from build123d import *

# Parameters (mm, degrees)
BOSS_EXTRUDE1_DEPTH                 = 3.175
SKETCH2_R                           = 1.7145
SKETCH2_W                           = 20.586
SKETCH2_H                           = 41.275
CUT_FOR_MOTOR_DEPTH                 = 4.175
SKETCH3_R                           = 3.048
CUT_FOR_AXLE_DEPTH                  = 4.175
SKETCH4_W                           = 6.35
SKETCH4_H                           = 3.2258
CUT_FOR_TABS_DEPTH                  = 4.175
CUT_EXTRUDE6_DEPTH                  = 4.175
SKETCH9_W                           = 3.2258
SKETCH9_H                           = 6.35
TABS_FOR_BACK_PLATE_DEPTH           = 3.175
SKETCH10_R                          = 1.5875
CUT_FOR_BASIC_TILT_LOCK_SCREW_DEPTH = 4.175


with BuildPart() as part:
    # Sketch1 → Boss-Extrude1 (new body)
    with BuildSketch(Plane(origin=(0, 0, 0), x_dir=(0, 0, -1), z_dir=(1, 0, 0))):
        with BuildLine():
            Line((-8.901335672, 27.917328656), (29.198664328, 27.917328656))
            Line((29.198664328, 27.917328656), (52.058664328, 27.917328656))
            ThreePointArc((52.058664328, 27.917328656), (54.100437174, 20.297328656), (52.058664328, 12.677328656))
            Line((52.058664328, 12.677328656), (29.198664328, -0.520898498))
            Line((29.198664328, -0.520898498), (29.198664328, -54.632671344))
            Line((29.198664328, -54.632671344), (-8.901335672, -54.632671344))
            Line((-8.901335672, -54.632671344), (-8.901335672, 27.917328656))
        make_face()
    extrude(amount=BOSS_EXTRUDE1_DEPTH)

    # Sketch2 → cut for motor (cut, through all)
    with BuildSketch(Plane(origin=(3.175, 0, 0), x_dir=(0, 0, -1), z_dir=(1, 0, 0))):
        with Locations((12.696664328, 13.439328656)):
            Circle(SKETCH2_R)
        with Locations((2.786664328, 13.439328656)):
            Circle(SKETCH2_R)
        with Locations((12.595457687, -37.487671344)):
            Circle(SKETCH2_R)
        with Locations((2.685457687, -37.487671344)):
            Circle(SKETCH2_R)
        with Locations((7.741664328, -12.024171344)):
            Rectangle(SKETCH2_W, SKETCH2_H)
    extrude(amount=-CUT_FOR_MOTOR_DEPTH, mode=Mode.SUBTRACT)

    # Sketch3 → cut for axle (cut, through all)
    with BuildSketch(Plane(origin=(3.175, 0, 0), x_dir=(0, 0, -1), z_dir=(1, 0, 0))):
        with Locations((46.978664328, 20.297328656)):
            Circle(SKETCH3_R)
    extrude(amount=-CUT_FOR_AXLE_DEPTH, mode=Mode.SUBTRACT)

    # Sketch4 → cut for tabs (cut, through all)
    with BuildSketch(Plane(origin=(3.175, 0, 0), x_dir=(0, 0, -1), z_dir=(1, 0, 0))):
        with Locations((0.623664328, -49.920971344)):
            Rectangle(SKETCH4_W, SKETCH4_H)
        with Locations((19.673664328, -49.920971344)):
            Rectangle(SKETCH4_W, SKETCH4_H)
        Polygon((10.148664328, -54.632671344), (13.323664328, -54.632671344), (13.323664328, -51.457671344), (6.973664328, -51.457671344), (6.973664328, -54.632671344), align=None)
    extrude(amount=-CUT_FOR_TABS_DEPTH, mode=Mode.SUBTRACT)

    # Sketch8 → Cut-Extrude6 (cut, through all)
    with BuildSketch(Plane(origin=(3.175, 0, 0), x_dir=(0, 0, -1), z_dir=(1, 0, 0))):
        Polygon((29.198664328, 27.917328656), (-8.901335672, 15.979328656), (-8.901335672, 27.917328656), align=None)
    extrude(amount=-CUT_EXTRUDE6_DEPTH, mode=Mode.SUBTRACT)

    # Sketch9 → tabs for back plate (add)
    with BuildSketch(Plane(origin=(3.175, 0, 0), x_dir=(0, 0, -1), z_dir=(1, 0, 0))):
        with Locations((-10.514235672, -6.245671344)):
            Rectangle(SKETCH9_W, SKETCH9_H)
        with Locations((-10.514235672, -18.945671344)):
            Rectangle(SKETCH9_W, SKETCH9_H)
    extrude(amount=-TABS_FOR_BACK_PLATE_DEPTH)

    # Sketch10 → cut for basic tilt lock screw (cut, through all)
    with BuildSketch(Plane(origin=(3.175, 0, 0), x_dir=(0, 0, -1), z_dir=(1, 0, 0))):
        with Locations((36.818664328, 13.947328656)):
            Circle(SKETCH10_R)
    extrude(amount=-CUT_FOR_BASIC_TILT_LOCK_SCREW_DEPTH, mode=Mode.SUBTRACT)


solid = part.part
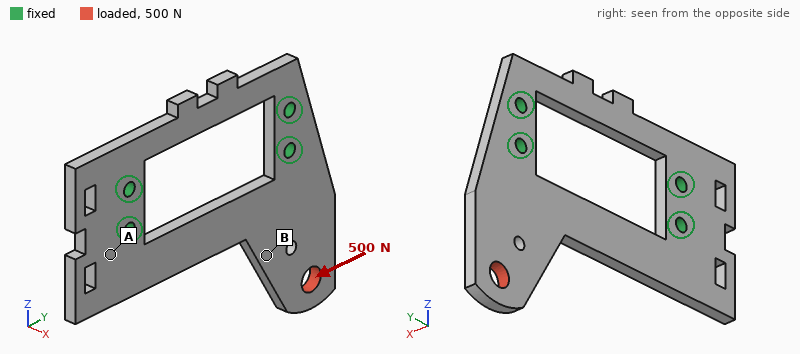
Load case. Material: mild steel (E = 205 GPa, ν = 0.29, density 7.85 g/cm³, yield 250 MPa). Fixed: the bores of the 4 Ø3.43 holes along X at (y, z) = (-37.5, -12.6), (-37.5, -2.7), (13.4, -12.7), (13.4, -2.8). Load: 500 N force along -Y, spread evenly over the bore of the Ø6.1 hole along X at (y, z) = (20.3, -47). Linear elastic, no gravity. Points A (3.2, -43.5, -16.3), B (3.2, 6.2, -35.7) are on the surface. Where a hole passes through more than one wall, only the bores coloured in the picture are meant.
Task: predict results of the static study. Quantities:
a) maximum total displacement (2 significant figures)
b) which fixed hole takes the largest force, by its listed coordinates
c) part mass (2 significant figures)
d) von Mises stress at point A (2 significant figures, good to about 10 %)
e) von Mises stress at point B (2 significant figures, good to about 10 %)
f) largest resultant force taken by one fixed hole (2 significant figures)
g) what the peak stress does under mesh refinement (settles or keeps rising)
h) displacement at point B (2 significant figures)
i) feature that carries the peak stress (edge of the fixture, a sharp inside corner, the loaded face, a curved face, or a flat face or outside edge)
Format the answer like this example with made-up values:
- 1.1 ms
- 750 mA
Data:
- 24 µm
- (-37.5, -12.6)
- 62 g
- 10 MPa
- 23 MPa
- 620 N
- keeps rising
- 11 µm
- a sharp inside corner
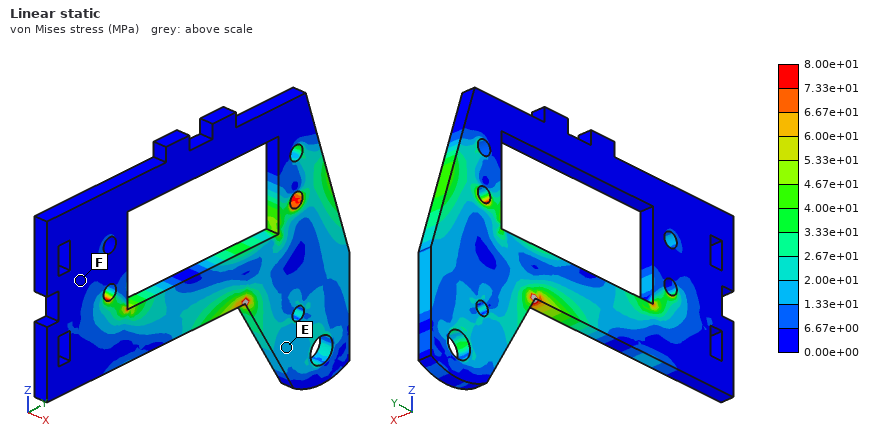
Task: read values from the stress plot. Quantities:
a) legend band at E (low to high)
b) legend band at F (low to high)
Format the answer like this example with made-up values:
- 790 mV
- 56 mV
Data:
- 1.33e+01 to 2.00e+01 MPa
- 0.00e+00 to 6.67e+00 MPa
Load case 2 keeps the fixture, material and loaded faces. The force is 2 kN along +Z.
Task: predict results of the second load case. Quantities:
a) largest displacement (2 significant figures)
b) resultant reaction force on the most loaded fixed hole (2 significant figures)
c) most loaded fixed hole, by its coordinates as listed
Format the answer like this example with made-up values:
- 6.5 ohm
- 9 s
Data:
- 23 µm
- 1.6 kN
- (13.4, -12.7)
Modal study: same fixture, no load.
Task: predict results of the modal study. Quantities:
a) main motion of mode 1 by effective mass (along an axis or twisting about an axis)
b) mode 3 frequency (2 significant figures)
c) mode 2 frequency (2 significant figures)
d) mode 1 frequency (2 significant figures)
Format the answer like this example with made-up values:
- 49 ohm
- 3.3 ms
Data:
- along X
- 4900 Hz
- 4300 Hz
- 1700 Hz
